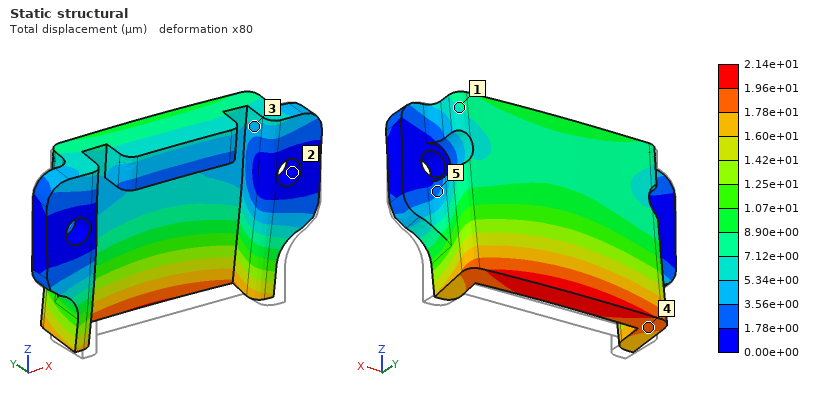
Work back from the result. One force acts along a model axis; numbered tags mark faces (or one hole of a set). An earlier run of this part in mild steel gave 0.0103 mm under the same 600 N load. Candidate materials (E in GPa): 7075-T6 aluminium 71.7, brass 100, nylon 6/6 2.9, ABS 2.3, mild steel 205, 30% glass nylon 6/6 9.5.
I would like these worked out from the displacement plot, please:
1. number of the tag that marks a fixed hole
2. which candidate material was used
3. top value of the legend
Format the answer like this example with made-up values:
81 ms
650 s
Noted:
2
brass
2.14e+01 µm
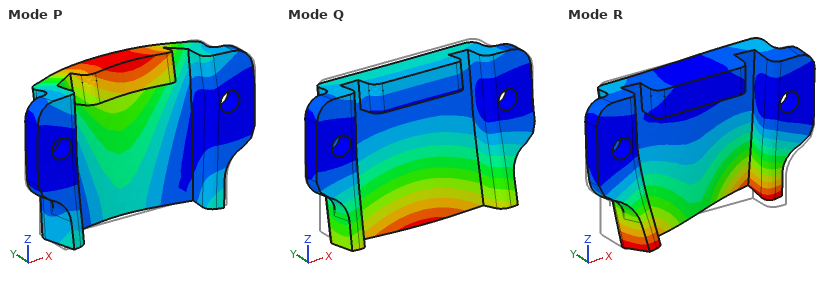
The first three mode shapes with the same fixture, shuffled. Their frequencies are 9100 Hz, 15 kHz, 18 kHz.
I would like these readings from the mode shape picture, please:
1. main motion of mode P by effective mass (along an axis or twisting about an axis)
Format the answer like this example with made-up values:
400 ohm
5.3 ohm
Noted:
along Y
